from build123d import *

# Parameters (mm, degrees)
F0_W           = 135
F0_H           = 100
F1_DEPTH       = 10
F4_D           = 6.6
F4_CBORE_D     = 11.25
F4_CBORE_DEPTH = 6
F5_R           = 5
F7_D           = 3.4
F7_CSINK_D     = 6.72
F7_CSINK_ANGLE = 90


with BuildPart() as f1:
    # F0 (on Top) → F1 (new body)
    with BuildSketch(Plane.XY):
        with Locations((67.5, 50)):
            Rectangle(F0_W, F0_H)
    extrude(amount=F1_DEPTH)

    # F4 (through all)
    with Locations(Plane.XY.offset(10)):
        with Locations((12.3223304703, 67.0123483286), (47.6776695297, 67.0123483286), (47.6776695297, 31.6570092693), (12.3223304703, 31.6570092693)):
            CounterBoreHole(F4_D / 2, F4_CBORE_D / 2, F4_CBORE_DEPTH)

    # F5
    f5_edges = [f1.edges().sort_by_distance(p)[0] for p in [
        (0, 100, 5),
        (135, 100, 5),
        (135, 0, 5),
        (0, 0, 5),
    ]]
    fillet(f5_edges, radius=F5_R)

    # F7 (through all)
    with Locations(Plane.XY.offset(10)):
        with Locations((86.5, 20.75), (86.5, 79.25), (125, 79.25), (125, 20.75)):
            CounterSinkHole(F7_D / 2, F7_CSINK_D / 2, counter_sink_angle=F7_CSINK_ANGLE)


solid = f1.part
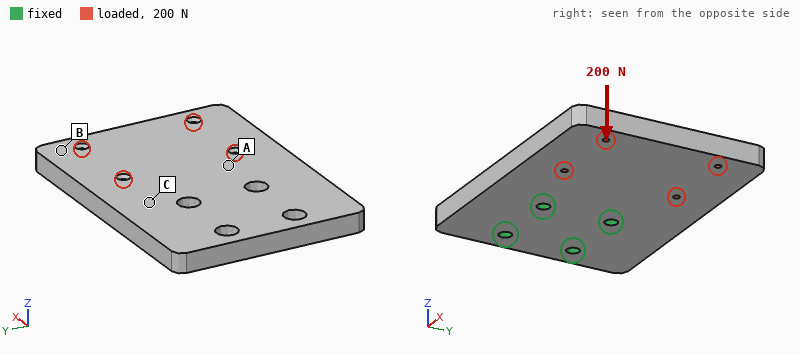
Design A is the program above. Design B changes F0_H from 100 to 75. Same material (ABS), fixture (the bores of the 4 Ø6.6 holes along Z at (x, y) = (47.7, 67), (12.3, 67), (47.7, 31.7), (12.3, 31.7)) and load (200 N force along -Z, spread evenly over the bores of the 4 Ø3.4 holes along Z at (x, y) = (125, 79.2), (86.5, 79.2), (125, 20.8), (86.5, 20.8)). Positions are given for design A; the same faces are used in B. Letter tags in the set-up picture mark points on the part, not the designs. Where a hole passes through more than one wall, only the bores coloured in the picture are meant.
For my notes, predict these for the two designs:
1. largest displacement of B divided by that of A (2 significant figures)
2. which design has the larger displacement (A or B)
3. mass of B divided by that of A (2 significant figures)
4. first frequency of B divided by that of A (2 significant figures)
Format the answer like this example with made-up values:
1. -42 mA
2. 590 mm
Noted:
1. 1.3
2. B
3. 0.74
4. 1.0
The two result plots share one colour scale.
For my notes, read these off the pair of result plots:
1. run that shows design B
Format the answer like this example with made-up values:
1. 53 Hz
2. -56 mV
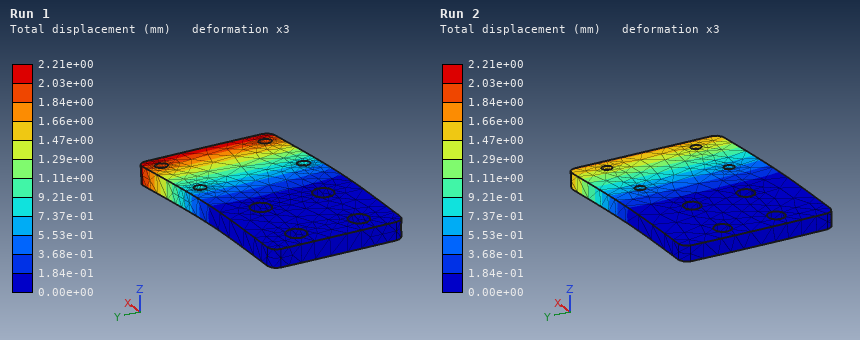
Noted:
1. Run 1
